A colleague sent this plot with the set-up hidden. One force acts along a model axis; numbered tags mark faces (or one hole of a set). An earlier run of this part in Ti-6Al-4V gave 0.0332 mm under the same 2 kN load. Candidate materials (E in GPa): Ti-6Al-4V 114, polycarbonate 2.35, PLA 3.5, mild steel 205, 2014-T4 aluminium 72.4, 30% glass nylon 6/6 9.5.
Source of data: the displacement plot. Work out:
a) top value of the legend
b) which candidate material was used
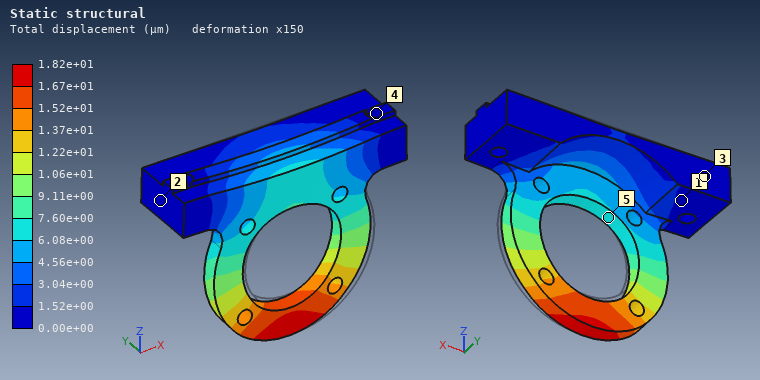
1.82e+01 µm
mild steel
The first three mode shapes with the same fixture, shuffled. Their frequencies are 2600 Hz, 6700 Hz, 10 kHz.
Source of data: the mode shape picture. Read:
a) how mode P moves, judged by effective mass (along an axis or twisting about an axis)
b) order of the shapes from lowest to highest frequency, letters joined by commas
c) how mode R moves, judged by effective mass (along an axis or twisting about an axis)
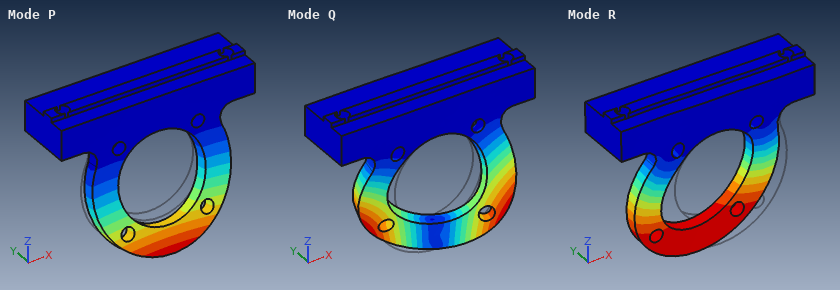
along Y
P, Q, R
along X
